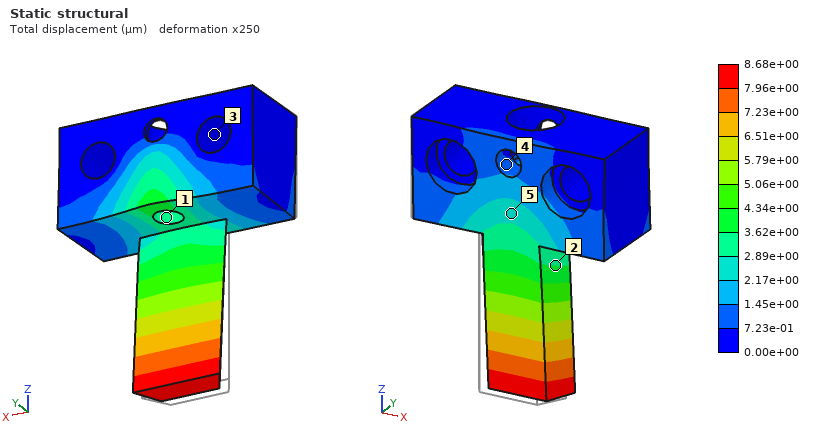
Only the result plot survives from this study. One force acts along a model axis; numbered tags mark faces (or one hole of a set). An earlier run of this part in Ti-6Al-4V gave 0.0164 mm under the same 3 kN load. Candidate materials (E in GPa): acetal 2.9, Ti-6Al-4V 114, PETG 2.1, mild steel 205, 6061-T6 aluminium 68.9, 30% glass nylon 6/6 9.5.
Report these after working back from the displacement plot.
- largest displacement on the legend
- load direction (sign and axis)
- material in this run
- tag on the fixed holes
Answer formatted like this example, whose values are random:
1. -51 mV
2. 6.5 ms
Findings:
1. 8.68e+00 µm
2. +Y
3. mild steel
4. 3
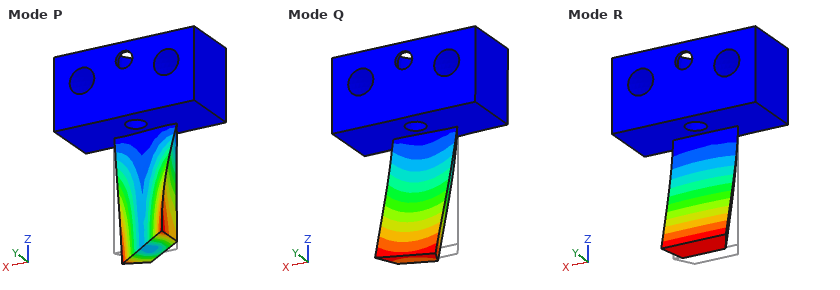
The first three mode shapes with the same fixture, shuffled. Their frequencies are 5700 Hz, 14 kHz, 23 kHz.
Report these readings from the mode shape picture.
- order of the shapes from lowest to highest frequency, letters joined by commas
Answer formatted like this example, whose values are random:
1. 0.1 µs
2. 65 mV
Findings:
1. R, Q, P
